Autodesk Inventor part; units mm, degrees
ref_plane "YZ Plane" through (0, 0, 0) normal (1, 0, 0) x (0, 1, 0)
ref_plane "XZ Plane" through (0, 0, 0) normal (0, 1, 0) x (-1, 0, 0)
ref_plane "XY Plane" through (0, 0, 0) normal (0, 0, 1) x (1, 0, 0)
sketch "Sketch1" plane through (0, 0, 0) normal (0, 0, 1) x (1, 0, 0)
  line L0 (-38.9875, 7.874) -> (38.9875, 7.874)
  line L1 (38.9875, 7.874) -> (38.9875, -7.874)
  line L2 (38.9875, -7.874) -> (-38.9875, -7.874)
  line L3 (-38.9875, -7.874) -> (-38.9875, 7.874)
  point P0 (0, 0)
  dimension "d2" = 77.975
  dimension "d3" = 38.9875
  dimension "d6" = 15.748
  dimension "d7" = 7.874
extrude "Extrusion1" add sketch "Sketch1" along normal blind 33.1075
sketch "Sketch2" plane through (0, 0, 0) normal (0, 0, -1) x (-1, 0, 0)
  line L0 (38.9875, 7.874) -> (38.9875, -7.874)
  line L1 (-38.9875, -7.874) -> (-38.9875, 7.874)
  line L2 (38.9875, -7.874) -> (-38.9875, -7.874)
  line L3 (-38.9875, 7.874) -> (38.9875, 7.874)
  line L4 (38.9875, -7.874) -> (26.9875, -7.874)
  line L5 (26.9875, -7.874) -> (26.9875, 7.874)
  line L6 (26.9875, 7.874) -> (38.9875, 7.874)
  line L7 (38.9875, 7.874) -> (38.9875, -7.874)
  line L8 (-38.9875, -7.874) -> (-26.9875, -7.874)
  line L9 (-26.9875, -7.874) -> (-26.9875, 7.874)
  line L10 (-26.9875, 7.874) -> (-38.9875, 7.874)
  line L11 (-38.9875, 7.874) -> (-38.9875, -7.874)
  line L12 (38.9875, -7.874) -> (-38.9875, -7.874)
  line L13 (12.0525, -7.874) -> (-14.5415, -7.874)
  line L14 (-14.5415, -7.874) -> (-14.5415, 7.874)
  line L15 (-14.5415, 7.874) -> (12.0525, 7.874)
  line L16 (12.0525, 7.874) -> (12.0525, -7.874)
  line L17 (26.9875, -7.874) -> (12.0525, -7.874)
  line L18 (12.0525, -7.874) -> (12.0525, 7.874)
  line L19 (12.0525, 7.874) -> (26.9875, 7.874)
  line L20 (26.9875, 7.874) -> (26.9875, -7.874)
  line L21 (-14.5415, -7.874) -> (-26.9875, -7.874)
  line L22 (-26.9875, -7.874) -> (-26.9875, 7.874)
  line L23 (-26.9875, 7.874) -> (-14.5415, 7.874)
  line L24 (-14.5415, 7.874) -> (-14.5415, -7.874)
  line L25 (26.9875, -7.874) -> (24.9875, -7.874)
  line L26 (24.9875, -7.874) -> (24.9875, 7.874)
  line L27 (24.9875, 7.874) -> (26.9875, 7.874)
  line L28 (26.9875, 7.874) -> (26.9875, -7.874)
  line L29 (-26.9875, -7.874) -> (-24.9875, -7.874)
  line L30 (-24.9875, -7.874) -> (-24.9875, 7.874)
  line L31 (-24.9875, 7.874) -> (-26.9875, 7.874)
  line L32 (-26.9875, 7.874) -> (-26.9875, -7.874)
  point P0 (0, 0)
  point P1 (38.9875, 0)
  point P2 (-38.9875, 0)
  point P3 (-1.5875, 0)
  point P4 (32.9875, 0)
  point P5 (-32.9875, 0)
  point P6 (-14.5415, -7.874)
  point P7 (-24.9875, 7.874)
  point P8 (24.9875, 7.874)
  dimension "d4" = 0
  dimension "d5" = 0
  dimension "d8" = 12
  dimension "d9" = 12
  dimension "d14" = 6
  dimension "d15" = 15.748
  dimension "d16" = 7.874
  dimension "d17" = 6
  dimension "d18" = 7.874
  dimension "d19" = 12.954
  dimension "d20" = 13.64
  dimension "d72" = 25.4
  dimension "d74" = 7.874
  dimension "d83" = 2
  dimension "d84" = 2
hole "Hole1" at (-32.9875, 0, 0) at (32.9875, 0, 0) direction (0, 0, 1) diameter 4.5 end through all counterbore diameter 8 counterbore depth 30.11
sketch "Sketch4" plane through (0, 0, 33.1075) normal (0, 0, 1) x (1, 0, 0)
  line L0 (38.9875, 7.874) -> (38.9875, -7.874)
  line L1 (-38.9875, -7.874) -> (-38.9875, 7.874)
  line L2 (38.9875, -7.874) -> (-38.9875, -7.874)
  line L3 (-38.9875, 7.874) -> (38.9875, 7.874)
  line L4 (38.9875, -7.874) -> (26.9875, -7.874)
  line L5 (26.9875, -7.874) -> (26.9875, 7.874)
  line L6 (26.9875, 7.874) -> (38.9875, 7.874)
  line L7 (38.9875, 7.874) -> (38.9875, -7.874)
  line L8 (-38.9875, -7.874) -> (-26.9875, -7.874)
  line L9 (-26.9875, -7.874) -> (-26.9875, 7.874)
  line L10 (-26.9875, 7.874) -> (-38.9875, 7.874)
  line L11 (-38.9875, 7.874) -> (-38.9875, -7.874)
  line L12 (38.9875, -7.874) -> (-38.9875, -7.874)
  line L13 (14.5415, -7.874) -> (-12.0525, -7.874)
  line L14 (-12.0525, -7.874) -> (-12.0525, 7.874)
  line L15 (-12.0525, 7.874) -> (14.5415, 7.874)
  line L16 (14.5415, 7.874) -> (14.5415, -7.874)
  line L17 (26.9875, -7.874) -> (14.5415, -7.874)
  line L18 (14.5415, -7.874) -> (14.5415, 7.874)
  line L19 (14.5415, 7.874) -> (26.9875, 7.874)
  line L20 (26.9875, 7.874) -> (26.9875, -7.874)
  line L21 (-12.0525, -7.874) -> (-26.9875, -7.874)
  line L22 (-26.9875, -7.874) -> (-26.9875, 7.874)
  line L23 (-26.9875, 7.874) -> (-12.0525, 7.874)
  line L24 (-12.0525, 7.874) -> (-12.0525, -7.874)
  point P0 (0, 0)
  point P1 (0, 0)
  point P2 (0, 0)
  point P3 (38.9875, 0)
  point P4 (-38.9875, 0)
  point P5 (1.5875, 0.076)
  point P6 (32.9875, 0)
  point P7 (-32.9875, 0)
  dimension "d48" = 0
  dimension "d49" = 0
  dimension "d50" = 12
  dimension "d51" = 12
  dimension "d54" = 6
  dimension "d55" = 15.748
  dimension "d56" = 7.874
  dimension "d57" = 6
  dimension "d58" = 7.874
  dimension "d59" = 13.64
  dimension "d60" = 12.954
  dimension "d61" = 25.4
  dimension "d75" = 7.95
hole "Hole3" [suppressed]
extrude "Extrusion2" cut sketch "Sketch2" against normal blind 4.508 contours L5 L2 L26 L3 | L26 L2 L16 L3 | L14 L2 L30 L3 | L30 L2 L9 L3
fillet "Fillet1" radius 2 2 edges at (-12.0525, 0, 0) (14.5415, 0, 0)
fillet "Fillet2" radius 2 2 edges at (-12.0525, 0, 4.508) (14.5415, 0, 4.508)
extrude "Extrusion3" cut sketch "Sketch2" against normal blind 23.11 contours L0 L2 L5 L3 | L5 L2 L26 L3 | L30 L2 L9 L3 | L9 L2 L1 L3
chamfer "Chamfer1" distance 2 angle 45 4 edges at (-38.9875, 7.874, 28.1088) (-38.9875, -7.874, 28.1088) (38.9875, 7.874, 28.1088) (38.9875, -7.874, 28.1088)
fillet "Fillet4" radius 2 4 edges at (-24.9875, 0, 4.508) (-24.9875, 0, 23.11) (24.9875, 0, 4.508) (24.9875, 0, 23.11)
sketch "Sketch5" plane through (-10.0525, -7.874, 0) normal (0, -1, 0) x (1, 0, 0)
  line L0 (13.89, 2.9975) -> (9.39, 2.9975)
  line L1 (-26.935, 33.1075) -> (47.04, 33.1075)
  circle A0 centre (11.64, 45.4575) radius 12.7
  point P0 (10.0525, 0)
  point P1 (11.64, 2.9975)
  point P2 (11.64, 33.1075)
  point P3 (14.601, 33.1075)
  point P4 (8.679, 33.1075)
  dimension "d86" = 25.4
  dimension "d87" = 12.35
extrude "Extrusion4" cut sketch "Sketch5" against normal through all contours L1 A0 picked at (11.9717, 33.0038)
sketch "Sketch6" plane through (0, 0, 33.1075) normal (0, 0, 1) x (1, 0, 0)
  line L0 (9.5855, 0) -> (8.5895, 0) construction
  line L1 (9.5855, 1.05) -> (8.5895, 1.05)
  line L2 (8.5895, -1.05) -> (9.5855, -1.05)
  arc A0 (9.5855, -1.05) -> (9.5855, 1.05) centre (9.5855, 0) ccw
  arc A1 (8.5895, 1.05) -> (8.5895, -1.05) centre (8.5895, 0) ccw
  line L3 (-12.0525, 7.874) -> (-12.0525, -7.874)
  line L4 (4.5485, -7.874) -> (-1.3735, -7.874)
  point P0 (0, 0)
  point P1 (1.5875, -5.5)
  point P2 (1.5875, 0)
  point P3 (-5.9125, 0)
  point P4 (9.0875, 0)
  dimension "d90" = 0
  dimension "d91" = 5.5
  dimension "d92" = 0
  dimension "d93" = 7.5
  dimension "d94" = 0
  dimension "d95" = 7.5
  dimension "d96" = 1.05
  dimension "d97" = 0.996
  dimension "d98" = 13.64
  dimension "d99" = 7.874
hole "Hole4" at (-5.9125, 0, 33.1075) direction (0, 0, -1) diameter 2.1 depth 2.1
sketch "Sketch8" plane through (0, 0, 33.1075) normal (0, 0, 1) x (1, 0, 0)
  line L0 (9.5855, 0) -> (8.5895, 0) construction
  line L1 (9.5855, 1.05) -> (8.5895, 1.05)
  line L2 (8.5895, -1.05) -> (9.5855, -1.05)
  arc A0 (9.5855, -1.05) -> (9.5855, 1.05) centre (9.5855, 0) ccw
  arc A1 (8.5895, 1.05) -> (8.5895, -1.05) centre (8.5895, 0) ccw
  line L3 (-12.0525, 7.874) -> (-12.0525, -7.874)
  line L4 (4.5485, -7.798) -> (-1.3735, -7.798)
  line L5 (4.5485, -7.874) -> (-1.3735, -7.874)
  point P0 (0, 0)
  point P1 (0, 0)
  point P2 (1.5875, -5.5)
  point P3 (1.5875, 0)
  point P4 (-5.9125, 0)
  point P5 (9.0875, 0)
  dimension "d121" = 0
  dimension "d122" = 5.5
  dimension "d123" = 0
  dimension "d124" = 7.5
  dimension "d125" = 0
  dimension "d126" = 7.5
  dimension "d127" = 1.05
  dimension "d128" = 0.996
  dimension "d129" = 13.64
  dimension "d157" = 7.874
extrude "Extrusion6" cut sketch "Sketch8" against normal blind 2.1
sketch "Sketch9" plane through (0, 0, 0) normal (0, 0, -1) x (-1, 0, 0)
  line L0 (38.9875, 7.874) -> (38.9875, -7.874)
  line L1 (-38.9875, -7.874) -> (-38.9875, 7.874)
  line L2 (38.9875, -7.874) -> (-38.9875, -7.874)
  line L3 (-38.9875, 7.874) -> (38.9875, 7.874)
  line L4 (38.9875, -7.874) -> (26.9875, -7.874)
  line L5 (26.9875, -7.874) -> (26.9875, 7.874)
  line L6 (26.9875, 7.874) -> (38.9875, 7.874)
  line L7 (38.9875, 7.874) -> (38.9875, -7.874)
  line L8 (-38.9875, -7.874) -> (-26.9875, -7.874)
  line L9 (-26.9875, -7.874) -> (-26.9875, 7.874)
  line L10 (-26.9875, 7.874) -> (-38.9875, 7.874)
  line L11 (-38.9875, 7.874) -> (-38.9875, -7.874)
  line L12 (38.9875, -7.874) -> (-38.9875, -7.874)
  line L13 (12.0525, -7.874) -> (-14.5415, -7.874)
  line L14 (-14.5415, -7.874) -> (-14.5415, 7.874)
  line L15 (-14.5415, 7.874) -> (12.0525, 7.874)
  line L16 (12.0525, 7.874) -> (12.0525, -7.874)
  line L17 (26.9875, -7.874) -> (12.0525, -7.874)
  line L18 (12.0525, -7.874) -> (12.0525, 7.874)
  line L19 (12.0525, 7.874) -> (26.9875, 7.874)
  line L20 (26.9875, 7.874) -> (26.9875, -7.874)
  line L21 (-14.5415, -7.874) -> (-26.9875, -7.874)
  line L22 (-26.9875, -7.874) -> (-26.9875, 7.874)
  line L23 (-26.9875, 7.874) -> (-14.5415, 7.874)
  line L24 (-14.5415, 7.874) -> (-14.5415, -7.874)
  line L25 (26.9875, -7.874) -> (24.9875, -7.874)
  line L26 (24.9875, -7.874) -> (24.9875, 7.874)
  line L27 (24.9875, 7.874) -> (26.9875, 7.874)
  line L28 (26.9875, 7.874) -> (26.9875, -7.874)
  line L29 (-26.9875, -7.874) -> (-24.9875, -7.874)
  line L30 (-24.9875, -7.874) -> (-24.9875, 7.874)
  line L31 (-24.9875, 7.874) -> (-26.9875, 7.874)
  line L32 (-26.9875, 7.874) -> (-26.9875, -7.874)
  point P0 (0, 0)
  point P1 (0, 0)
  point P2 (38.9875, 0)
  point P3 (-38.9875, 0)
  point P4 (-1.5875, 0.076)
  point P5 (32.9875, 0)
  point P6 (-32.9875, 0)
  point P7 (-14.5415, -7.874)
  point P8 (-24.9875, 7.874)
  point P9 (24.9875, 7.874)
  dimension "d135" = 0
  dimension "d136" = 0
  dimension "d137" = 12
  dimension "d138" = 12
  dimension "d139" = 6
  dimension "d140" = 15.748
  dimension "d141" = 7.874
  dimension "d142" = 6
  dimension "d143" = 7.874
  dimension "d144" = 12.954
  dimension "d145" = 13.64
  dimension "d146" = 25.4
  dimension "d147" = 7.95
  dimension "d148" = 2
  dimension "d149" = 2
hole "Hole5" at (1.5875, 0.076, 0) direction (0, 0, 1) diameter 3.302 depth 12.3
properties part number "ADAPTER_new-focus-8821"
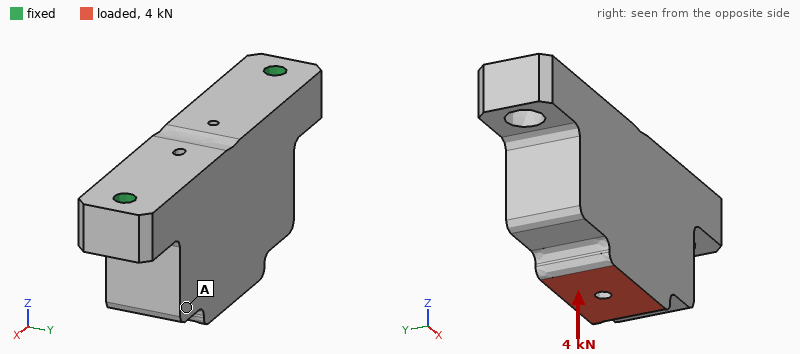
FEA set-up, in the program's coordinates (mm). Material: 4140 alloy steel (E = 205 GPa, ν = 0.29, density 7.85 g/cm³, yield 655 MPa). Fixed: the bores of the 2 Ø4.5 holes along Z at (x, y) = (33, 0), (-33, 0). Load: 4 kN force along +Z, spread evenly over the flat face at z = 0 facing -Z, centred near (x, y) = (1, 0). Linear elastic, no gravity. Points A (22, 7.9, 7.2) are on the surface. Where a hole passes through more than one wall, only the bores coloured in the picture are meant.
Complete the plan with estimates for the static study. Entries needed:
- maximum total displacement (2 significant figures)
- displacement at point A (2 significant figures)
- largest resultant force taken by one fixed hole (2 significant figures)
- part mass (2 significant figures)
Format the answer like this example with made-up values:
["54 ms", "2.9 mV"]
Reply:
["7.7 µm", "6.2 µm", "2.6 kN", "220 g"]
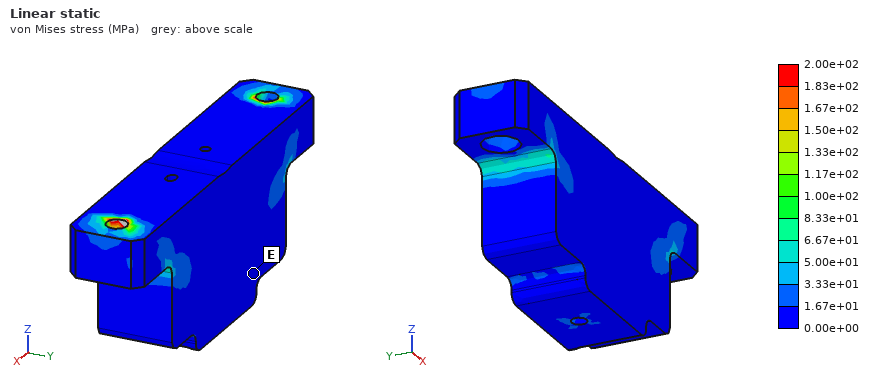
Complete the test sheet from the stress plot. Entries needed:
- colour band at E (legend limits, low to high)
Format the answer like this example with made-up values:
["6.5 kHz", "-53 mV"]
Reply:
["0.00e+00 to 1.67e+01 MPa"]
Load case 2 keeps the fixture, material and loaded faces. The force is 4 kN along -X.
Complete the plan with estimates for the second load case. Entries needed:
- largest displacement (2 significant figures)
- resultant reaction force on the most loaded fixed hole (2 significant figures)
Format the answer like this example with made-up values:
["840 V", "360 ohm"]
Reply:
["8.3 µm", "2.8 kN"]
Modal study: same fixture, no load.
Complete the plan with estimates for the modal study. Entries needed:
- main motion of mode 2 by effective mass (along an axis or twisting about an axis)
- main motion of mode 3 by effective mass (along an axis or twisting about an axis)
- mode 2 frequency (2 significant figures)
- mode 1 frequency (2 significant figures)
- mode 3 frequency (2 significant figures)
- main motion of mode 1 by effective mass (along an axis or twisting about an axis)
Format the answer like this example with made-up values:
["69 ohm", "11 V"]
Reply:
["along Z", "along Y", "9000 Hz", "2400 Hz", "11 kHz", "along Y"]
